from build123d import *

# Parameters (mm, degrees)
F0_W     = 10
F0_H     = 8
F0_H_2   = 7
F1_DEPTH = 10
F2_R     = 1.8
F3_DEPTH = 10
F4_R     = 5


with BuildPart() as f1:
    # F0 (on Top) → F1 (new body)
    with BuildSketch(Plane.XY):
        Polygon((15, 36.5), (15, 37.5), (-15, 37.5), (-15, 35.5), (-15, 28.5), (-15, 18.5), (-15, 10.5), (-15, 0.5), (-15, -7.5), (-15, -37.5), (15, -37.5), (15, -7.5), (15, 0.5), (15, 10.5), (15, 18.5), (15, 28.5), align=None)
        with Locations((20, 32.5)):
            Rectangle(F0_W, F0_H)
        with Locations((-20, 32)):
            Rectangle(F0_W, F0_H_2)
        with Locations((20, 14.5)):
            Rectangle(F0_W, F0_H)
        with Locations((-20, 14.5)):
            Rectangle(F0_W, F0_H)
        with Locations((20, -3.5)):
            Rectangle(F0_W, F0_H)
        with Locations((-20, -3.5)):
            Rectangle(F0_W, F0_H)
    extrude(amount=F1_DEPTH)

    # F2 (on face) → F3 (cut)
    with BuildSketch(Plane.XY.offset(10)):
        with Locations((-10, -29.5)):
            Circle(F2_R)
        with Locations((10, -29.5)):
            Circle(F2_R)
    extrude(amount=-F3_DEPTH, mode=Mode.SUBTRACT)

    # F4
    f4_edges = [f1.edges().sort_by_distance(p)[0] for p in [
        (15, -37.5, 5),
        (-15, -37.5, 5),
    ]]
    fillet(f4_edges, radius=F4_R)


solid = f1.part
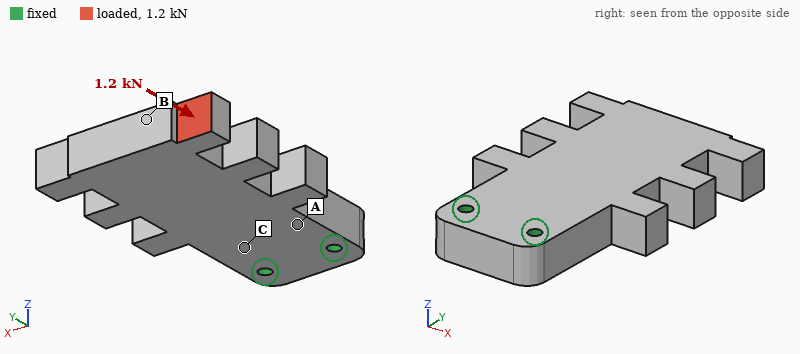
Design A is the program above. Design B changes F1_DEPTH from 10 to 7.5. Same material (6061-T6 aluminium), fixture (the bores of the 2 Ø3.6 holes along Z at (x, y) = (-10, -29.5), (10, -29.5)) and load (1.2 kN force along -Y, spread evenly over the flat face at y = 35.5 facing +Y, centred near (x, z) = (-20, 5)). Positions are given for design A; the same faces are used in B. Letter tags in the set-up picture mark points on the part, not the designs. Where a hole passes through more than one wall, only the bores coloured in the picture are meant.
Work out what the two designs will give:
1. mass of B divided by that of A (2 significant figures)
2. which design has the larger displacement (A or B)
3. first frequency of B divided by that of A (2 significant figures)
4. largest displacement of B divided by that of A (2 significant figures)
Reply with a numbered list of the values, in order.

1. 0.75
2. B
3. 0.76
4. 1.4
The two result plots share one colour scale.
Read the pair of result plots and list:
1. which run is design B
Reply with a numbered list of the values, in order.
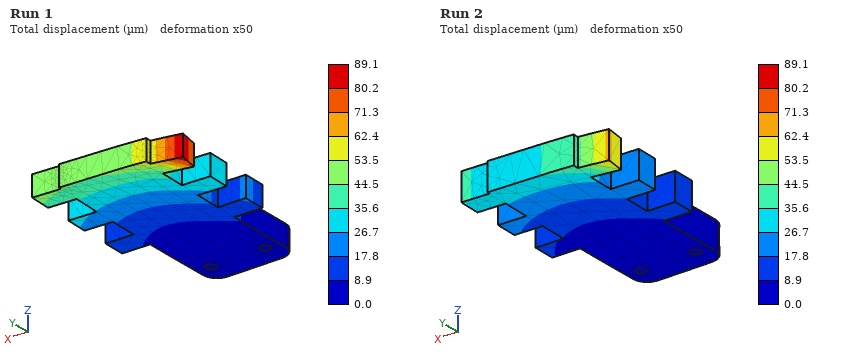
1. Run 1
